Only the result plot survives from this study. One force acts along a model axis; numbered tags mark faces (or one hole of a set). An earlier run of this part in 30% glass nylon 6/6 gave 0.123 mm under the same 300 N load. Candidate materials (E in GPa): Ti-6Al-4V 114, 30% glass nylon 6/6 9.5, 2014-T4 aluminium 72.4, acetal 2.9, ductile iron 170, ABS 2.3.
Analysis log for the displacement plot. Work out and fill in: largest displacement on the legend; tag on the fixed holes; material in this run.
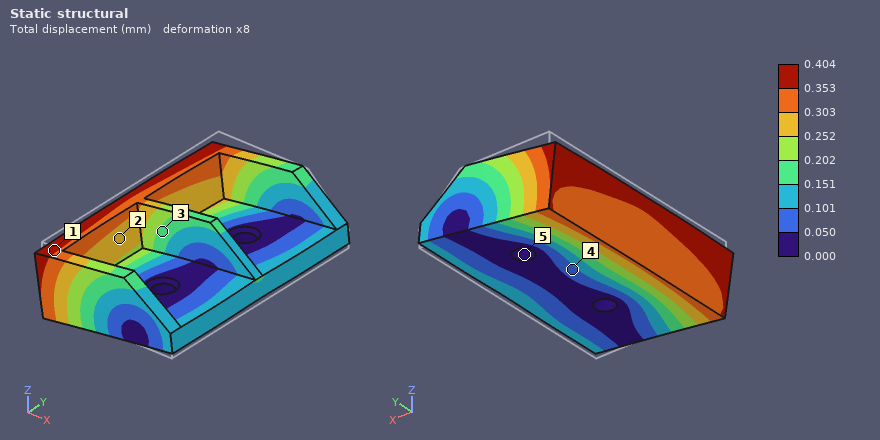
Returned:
0.404 mm
5
acetal
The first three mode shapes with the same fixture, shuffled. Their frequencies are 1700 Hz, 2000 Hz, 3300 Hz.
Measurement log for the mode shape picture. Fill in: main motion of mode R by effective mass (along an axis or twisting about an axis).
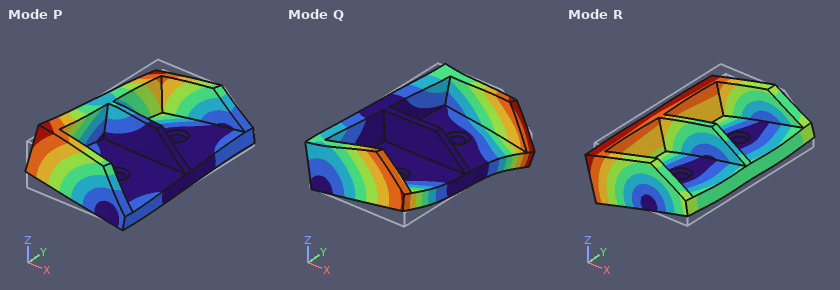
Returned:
along Z
